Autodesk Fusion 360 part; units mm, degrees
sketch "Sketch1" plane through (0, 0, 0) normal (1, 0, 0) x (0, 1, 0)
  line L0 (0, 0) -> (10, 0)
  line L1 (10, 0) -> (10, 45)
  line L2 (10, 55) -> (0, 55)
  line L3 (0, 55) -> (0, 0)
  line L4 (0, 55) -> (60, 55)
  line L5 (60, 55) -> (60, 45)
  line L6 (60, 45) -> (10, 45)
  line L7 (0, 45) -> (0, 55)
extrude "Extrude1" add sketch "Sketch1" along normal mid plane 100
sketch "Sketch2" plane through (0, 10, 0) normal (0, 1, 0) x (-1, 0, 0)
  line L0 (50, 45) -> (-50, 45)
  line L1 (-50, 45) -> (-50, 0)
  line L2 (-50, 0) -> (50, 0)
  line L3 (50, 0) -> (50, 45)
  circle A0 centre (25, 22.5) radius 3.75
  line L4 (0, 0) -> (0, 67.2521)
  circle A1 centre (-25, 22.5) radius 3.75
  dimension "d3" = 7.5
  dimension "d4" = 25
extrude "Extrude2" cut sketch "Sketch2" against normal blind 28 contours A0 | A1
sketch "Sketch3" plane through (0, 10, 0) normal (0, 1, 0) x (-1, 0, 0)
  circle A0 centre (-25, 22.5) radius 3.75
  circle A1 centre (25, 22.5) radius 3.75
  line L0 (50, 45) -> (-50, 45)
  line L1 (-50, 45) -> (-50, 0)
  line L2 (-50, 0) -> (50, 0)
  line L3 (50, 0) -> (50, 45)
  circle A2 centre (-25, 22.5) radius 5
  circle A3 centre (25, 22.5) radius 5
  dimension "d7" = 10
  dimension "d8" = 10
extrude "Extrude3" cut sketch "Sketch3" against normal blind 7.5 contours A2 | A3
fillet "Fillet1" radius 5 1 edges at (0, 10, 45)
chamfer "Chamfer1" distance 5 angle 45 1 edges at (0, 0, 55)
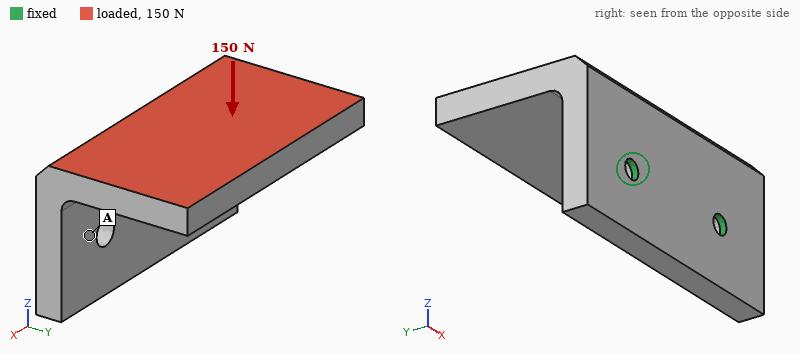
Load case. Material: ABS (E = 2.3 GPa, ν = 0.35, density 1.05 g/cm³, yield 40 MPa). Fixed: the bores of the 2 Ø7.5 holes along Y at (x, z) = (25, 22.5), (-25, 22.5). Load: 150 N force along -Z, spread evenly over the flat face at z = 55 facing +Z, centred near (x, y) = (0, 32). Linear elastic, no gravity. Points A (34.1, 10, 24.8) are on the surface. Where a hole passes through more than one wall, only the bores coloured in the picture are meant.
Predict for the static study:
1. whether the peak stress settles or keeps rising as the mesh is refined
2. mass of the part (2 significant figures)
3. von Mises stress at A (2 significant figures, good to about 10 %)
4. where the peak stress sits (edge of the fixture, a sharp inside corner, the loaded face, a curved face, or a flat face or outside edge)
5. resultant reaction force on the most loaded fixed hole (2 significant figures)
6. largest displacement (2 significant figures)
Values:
keeps rising
110 g
3.5 MPa
edge of the fixture
75 N
1.3 mm
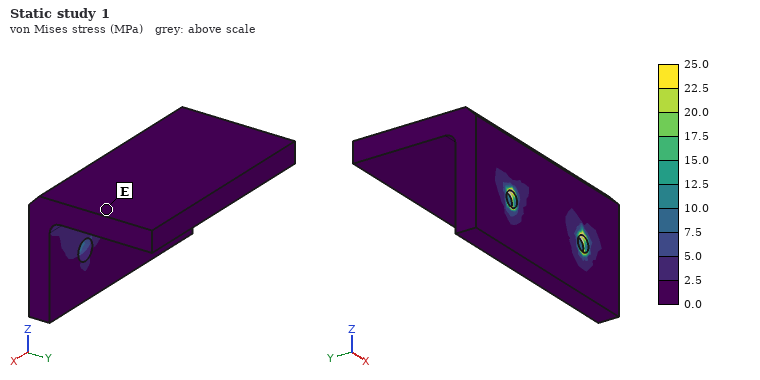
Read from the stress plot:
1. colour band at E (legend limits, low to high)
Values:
0.0 to 2.5 MPa
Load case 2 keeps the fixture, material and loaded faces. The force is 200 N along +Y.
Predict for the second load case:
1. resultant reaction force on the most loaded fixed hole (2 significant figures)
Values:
100 N
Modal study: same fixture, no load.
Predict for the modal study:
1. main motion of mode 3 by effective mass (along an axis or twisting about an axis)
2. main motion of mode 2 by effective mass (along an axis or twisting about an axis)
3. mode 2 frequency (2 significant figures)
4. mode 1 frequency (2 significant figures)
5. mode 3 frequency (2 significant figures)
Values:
along Y
along X
620 Hz
240 Hz
1100 Hz
